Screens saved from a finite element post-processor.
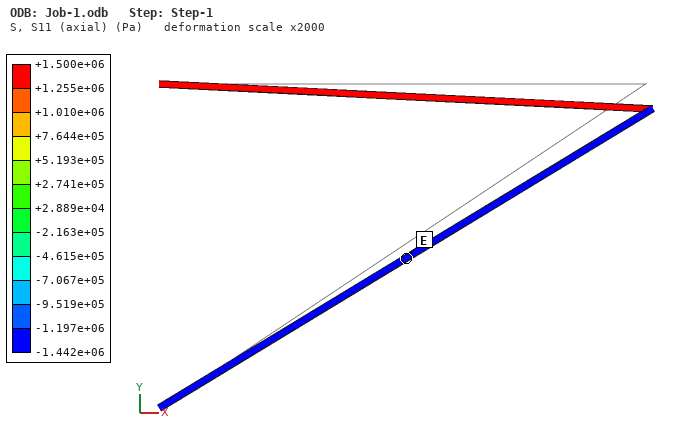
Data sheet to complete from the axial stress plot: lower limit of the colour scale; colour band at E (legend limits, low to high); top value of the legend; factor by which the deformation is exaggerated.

-1.442e+06 Pa
-1.442e+06 to -1.197e+06 Pa
+1.500e+06 Pa
2000
